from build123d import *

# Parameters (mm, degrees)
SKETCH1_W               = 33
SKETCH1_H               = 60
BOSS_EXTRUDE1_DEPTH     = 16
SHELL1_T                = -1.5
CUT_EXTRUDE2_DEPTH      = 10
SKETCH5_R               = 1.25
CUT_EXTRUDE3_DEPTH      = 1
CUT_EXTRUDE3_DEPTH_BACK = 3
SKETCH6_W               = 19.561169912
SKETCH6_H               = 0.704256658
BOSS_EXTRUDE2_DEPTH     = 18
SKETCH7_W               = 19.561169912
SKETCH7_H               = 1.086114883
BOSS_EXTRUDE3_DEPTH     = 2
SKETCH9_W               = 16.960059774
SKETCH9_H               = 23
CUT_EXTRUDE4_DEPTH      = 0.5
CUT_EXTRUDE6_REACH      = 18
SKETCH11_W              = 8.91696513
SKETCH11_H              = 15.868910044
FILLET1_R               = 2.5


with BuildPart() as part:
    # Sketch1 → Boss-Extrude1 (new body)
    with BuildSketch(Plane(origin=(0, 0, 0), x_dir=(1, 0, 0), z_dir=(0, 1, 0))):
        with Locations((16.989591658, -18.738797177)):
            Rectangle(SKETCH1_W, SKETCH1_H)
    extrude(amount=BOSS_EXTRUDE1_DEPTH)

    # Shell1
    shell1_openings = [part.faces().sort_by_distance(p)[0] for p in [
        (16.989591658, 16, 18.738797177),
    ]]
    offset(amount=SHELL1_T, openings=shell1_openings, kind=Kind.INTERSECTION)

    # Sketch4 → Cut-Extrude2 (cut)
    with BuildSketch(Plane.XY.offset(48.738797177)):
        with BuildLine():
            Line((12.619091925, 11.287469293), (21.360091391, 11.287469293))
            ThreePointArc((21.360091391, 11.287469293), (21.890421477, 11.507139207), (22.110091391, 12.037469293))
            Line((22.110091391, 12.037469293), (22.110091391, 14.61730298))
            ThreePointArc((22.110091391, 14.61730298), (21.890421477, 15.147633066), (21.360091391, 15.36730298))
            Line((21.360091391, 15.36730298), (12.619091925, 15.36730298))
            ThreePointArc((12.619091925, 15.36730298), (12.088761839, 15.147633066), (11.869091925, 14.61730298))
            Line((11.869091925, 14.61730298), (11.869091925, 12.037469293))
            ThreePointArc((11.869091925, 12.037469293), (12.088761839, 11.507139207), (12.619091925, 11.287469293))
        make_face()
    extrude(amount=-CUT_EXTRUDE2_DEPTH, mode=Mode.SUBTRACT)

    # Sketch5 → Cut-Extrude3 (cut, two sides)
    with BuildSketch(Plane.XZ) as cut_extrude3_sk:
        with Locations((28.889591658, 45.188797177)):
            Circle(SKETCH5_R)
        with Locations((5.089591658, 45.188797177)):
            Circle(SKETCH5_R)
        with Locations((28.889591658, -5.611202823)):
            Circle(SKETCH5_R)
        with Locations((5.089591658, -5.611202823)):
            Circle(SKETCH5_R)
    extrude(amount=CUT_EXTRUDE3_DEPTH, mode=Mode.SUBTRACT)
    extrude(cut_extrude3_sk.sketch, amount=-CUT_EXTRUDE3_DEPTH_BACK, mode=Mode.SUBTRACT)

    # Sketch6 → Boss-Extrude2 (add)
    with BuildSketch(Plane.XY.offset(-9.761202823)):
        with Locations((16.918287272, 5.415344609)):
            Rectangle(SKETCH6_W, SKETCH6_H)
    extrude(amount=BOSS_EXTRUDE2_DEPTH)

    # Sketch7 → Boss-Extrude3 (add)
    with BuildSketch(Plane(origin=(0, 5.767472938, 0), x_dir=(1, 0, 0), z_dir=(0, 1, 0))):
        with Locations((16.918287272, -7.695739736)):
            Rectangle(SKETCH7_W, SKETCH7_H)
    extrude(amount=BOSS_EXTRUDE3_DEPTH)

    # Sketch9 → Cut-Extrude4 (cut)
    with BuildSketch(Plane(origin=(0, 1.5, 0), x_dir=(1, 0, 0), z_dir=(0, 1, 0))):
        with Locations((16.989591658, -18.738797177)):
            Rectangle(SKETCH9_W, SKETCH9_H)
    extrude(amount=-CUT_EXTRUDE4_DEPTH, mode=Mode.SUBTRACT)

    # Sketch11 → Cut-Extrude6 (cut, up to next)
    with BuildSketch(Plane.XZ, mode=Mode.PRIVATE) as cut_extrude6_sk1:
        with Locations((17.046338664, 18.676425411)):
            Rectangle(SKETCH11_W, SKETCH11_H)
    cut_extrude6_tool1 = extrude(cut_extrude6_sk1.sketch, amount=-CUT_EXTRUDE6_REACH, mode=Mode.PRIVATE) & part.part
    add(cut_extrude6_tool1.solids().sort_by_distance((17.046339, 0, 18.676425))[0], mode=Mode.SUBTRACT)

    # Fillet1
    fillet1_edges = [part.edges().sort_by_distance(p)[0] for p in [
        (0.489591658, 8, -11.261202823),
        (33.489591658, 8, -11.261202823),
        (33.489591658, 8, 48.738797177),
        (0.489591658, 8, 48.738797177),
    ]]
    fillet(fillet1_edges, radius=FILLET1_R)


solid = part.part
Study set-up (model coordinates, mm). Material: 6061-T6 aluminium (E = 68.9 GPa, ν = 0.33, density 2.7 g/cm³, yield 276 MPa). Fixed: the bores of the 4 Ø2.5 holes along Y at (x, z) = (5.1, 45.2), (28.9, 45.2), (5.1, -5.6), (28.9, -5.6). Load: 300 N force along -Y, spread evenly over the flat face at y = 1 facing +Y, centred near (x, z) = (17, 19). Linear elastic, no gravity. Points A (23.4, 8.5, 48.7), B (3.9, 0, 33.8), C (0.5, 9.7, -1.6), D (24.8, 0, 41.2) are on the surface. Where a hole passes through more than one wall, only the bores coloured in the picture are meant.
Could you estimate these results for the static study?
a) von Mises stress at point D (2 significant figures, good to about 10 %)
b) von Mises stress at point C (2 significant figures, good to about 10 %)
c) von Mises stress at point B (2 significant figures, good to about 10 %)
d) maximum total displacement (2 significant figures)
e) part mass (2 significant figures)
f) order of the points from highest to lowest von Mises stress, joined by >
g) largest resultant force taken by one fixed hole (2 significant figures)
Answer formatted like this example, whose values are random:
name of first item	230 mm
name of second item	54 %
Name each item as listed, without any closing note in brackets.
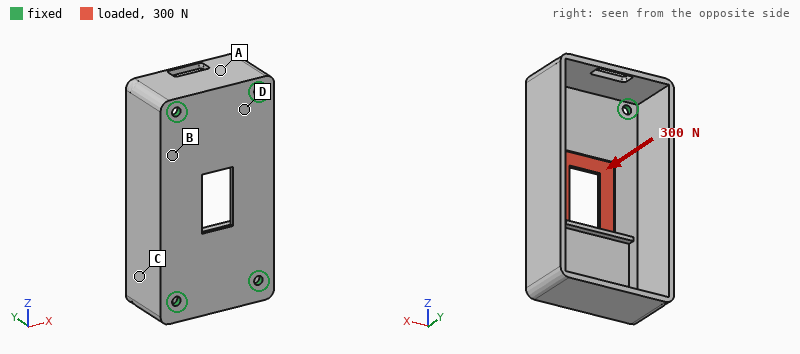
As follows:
von Mises stress at point D	32 MPa
von Mises stress at point C	20 MPa
von Mises stress at point B	47 MPa
maximum total displacement	0.18 mm
part mass	18 g
order of the points from highest to lowest von Mises stress, joined by >	B > D > C > A
largest resultant force taken by one fixed hole	86 N
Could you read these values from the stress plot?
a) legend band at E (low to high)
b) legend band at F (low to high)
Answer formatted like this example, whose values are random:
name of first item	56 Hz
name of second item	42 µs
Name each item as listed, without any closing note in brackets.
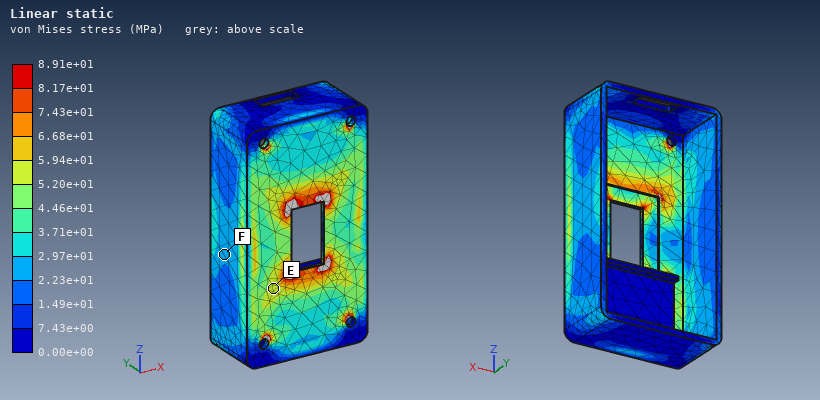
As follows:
legend band at E	5.20e+01 to 5.94e+01 MPa
legend band at F	2.23e+01 to 2.97e+01 MPa
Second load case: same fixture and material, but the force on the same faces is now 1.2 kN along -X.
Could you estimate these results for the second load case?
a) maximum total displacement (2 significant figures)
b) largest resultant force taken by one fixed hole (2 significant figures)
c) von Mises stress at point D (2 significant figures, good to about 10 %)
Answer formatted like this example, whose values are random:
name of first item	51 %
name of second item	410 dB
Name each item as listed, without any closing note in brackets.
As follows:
maximum total displacement	18 µm
largest resultant force taken by one fixed hole	380 N
von Mises stress at point D	27 MPa
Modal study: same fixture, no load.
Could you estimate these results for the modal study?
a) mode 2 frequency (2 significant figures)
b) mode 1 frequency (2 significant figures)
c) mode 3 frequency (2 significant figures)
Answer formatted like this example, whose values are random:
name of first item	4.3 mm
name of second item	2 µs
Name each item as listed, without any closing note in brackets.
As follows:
mode 2 frequency	3500 Hz
mode 1 frequency	1400 Hz
mode 3 frequency	3900 Hz
